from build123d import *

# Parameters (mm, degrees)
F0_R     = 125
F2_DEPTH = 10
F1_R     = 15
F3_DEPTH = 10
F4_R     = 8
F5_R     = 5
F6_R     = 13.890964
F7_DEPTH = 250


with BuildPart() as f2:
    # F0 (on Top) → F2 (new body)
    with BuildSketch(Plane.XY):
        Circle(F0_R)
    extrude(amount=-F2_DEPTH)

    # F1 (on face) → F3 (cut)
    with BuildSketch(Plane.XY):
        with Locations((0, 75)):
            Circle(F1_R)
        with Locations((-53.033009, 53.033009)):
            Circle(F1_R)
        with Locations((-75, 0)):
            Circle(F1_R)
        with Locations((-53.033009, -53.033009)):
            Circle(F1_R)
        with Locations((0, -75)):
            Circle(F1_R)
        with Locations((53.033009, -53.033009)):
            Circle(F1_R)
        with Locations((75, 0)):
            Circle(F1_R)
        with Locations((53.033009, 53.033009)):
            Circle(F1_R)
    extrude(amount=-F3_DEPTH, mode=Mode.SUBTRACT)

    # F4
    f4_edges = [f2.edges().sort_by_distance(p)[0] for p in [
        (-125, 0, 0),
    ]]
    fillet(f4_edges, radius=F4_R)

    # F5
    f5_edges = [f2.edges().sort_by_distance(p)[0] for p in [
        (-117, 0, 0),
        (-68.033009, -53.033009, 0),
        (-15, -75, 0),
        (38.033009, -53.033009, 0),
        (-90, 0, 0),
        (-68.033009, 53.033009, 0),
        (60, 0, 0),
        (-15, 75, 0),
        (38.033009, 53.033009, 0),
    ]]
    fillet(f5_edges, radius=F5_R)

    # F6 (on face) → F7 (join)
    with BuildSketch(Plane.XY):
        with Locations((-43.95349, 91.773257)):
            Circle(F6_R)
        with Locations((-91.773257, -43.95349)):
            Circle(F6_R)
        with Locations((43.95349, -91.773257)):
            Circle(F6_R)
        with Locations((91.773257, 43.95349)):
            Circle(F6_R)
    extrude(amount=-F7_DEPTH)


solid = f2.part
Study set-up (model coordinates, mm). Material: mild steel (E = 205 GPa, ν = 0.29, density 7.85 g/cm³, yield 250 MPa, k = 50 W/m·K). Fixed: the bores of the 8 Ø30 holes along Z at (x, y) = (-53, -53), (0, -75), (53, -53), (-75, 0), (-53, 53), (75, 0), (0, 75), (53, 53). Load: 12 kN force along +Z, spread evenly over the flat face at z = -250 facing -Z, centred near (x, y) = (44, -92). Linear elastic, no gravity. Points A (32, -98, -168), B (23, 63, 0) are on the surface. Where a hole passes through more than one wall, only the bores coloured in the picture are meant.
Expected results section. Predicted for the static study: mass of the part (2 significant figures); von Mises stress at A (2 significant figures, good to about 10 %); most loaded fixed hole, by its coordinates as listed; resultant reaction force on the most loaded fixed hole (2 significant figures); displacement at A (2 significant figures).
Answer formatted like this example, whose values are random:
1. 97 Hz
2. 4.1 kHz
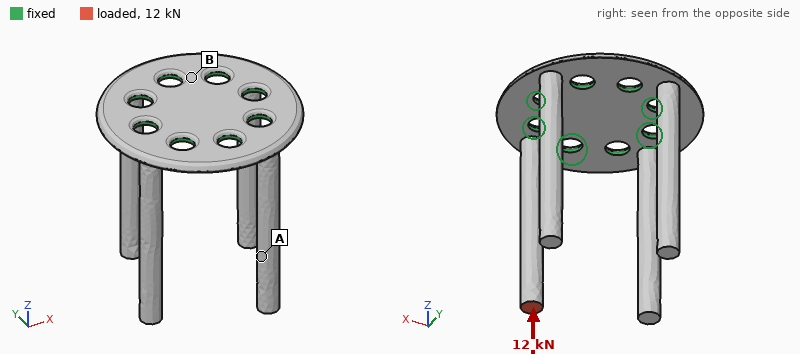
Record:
1. 7.9 kg
2. 20 MPa
3. (53, -53)
4. 7.9 kN
5. 0.38 mm
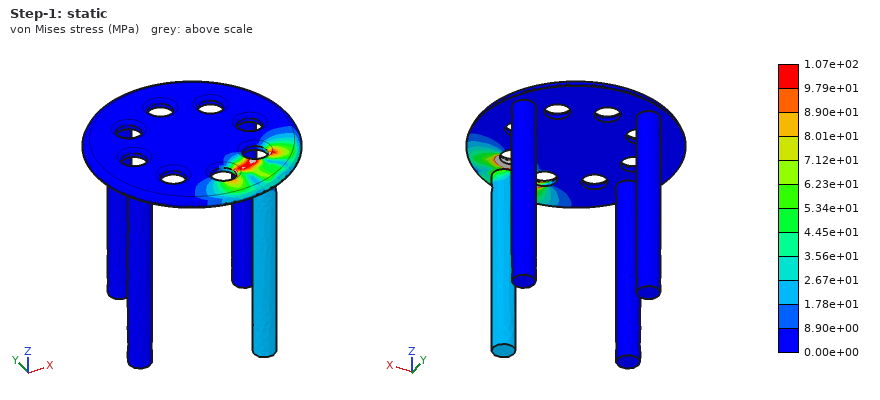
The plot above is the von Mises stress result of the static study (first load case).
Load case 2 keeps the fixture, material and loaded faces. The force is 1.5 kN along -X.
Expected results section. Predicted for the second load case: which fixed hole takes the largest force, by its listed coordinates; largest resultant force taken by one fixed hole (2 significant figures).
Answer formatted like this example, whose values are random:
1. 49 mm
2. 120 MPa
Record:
1. (53, -53)
2. 7.7 kN
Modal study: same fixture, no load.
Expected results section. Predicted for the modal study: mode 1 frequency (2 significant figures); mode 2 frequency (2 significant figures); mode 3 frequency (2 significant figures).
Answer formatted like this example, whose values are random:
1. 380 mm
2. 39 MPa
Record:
1. 220 Hz
2. 220 Hz
3. 220 Hz
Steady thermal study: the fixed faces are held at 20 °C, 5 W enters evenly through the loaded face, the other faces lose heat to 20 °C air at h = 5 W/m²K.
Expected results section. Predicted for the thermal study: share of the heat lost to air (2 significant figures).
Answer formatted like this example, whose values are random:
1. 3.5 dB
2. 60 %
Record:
1. 36 %
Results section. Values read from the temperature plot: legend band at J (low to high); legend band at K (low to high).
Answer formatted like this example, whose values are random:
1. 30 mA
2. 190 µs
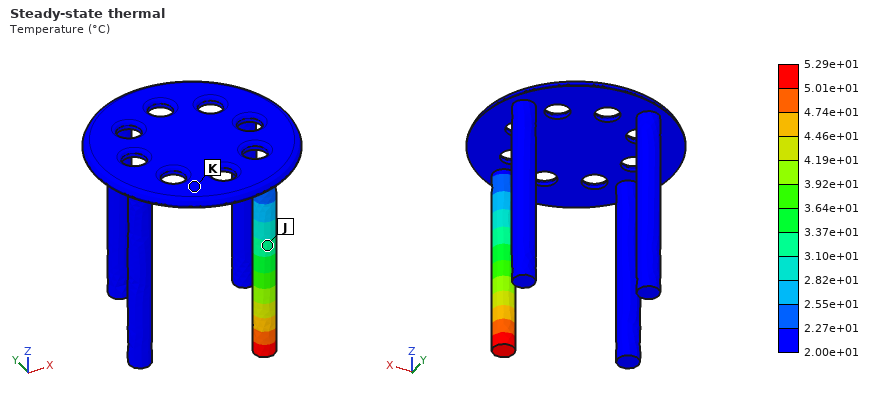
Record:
1. 3.10e+01 to 3.37e+01 °C
2. 2.00e+01 to 2.27e+01 °C
